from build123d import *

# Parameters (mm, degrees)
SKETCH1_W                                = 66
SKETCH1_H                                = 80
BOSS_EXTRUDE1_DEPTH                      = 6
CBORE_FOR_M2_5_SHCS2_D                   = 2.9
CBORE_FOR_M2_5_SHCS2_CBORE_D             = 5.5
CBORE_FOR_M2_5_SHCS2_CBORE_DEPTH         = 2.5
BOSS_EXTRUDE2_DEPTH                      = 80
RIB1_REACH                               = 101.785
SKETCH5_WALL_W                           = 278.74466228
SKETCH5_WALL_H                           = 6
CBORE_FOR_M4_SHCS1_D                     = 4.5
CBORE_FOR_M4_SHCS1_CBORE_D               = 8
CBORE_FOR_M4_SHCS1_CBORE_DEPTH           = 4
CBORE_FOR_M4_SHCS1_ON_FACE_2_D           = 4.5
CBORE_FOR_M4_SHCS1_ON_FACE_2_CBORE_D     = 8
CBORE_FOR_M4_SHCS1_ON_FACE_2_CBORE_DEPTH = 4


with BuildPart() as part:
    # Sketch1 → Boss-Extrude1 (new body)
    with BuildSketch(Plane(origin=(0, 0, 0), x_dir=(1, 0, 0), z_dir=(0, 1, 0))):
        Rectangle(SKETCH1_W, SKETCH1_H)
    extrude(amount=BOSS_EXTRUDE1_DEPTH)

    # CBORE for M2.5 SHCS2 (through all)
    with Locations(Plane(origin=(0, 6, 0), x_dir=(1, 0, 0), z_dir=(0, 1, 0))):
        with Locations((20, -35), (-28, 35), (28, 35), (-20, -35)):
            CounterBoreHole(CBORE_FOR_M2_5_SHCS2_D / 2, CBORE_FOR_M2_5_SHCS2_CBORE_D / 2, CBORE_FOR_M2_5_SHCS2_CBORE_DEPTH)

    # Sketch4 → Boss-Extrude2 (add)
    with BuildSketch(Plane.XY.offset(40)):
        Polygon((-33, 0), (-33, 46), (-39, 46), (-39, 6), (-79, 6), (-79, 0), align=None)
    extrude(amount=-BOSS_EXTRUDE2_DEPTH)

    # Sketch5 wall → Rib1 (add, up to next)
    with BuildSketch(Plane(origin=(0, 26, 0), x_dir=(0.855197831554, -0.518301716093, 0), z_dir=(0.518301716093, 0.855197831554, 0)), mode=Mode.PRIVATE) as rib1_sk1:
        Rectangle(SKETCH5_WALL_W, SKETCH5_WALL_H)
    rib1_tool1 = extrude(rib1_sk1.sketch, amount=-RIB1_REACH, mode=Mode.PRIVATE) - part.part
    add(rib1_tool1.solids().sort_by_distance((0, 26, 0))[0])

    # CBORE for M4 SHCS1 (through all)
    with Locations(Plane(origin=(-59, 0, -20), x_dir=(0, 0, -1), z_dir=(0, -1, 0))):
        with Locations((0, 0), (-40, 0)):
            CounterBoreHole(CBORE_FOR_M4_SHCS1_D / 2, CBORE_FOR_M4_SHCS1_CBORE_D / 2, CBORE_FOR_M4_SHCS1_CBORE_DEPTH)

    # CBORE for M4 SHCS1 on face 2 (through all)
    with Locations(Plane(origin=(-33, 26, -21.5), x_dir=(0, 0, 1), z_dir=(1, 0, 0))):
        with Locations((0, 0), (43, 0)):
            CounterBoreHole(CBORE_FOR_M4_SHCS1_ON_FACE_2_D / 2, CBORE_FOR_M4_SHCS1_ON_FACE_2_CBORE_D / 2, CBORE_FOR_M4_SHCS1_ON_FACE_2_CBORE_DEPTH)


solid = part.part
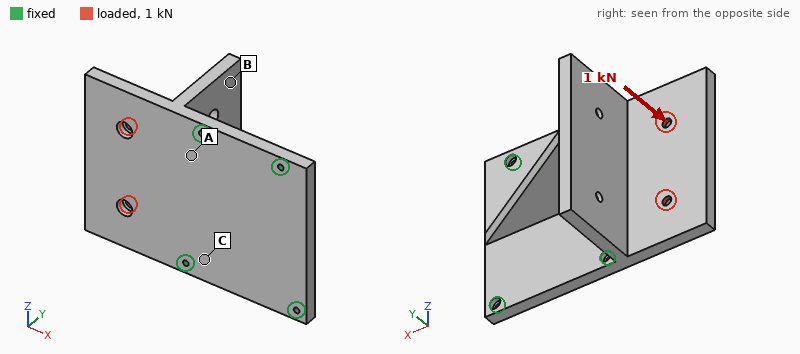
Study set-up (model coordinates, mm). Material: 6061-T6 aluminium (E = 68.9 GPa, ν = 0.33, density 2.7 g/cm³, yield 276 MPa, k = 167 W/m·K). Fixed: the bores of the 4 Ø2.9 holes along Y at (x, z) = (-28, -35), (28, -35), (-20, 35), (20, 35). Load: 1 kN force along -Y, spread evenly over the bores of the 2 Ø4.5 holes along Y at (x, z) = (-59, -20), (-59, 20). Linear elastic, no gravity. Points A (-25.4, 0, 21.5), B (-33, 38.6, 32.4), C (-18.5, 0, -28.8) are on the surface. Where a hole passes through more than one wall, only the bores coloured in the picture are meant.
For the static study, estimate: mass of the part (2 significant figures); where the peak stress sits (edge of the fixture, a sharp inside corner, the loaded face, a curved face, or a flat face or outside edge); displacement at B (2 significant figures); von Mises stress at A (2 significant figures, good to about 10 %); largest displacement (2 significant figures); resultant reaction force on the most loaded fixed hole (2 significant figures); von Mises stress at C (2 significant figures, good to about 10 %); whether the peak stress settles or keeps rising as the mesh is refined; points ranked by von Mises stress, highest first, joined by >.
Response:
210 g
edge of the fixture
0.093 mm
24 MPa
0.26 mm
1.0 kN
13 MPa
keeps rising
A > C > B
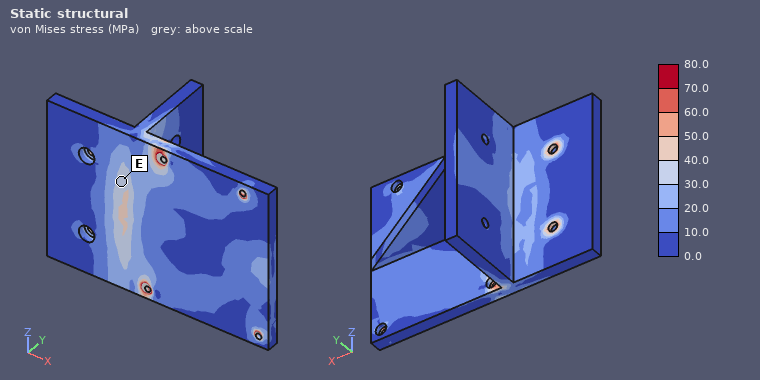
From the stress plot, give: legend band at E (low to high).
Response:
30.0 to 40.0 MPa
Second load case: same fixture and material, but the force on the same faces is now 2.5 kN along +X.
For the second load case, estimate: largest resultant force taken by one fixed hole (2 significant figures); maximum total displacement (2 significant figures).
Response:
880 N
58 µm
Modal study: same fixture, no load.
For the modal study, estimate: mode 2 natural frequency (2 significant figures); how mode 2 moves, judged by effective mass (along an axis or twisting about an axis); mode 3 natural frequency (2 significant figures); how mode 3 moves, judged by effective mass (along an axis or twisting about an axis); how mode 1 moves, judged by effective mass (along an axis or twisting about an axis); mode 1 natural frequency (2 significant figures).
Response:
2800 Hz
twisting about X
3500 Hz
along Y
along Y
1500 Hz
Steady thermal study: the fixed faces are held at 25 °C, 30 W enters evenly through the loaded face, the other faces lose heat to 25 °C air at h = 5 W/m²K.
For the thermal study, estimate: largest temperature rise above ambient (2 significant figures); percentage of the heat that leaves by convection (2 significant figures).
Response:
25 K
4.2 %
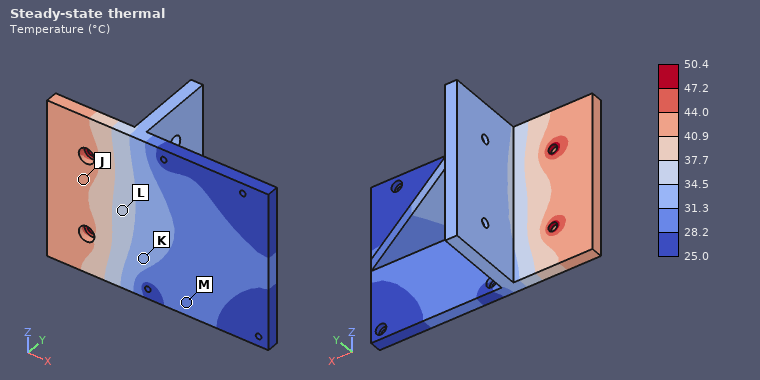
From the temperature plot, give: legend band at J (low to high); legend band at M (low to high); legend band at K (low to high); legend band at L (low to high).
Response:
40.9 to 44.0 °C
28.2 to 31.3 °C
31.3 to 34.5 °C
34.5 to 37.7 °C
